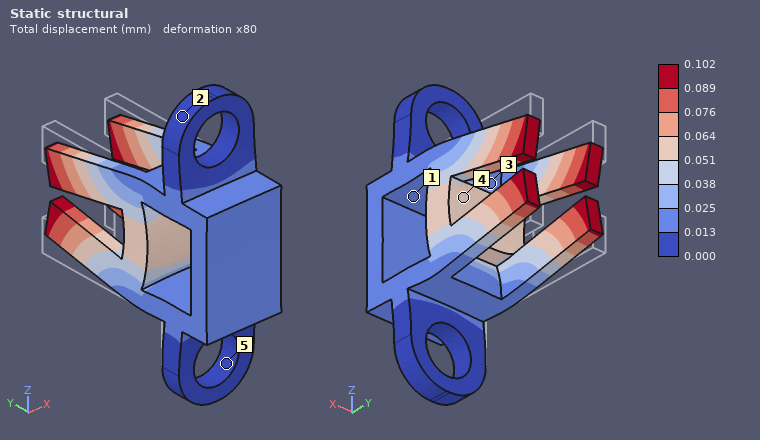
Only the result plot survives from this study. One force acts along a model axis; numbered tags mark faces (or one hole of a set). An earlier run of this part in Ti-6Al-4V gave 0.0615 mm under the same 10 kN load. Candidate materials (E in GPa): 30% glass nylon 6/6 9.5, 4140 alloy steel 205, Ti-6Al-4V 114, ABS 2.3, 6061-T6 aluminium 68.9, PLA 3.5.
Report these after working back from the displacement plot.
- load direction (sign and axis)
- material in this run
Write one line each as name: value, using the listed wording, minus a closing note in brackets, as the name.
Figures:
load direction: -Y
material in this run: 6061-T6 aluminium
